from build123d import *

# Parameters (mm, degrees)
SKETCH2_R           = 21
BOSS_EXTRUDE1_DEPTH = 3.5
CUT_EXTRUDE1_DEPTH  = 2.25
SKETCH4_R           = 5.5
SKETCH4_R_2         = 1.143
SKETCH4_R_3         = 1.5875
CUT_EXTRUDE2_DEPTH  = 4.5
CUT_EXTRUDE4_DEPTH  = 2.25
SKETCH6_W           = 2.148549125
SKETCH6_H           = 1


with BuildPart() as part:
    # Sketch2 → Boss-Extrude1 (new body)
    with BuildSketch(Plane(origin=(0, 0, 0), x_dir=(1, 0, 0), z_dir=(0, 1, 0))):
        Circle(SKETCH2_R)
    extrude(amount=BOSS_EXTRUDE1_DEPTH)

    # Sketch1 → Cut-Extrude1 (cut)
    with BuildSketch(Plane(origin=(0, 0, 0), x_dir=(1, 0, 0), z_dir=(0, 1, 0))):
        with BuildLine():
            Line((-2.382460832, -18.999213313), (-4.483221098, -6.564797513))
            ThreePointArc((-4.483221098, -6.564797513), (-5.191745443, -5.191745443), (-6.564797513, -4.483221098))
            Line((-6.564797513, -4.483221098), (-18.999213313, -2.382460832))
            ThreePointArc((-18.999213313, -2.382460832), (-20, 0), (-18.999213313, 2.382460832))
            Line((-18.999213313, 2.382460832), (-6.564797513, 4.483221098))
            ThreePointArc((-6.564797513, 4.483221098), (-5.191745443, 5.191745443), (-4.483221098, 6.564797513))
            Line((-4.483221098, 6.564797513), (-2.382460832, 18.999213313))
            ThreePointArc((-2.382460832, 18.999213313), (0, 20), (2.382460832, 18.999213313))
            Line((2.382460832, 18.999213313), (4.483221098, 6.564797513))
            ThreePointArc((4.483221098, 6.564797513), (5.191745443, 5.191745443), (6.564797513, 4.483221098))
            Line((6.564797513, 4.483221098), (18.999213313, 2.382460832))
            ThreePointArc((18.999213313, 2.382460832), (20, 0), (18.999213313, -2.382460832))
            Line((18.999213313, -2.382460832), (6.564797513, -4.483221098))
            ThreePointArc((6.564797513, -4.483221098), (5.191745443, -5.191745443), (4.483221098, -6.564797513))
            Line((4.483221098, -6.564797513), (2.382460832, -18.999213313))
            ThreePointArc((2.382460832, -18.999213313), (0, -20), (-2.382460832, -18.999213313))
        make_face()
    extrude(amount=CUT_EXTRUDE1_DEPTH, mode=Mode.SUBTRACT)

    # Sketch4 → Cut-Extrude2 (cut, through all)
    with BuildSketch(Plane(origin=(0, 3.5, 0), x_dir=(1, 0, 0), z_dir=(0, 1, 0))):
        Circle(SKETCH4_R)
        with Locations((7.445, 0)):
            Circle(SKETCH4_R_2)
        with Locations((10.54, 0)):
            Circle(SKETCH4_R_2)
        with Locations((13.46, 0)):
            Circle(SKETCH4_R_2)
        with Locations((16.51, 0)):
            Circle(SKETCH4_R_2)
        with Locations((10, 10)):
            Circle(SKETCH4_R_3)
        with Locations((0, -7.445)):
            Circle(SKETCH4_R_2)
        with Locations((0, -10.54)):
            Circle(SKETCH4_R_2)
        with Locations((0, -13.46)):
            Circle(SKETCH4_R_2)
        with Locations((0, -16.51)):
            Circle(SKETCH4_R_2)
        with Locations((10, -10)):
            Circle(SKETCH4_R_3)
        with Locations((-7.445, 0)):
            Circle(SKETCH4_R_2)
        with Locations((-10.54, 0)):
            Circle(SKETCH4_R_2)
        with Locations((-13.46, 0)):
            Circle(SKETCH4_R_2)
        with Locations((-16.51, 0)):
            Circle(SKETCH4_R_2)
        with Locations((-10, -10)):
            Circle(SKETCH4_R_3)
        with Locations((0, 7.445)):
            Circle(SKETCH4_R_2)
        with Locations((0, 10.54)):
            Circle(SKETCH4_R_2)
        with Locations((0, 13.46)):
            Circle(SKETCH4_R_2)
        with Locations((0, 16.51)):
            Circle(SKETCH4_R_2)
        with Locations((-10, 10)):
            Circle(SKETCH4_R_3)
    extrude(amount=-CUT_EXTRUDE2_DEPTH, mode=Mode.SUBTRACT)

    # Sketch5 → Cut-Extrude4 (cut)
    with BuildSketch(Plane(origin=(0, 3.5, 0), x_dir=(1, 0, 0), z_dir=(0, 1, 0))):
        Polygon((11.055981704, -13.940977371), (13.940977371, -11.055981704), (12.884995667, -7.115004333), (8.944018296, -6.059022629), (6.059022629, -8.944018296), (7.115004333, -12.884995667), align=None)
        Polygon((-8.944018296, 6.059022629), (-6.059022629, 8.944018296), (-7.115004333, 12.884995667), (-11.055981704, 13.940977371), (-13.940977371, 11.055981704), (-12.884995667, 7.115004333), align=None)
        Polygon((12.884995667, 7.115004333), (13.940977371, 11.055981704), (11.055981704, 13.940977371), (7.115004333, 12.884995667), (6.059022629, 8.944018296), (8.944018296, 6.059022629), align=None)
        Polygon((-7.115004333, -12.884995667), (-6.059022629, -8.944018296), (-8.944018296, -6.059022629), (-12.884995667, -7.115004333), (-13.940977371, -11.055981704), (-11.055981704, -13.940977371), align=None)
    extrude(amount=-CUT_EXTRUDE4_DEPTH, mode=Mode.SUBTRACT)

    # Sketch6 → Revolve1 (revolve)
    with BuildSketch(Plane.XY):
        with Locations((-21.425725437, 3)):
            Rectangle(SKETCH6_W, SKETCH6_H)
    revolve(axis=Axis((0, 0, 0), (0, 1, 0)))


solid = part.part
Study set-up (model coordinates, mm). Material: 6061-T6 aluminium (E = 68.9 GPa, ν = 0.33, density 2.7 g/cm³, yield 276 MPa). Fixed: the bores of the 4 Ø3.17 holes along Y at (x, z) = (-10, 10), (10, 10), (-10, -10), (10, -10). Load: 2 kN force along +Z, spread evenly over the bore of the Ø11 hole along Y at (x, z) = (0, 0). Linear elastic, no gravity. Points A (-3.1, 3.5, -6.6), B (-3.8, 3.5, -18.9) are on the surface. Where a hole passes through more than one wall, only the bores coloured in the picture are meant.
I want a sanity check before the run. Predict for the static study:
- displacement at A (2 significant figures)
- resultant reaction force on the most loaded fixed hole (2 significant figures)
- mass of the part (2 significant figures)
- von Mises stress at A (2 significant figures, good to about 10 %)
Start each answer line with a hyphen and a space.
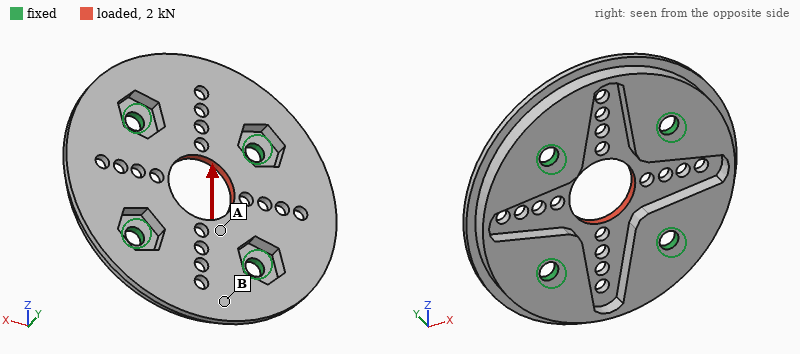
- 19 µm
- 510 N
- 8.8 g
- 48 MPa
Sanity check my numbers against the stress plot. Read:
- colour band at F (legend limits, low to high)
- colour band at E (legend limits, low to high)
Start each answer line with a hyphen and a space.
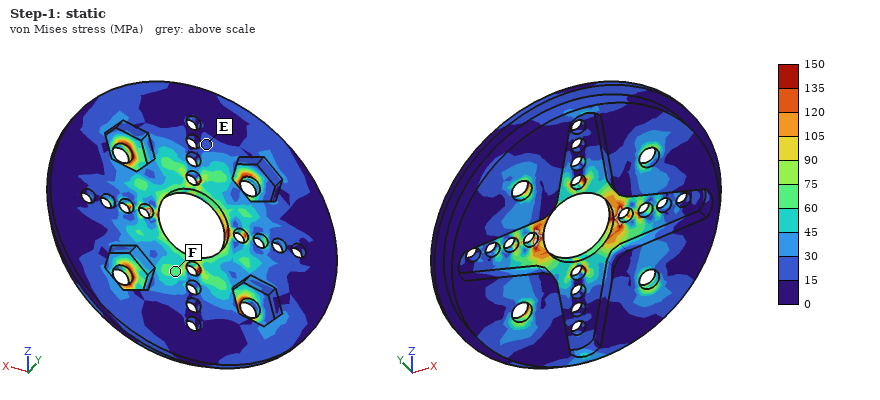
- 60 to 75 MPa
- 15 to 30 MPa
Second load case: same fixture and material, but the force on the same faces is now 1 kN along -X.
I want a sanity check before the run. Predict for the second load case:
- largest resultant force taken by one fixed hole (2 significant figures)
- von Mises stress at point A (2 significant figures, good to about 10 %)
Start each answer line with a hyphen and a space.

- 250 N
- 24 MPa
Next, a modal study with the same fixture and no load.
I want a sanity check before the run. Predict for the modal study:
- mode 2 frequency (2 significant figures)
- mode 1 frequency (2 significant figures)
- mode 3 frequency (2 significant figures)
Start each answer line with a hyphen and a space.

- 14 kHz
- 12 kHz
- 14 kHz
